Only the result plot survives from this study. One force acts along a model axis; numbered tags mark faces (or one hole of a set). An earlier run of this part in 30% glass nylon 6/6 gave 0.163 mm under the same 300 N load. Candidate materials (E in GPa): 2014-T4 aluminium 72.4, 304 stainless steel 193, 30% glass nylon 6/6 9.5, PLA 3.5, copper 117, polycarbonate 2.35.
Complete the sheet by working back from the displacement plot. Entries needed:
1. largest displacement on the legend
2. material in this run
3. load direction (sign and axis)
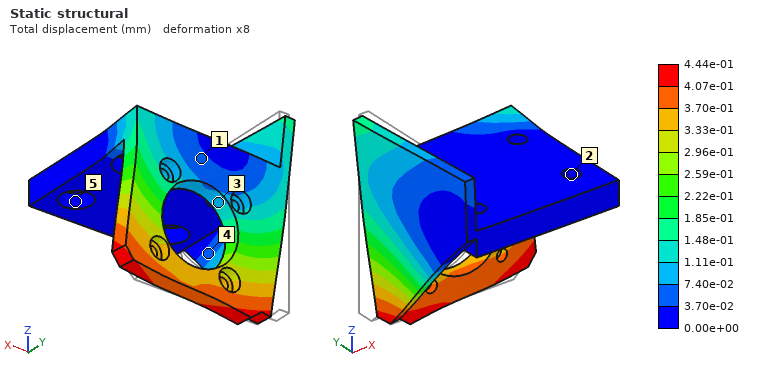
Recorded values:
4.44e-01 mm
PLA
+X
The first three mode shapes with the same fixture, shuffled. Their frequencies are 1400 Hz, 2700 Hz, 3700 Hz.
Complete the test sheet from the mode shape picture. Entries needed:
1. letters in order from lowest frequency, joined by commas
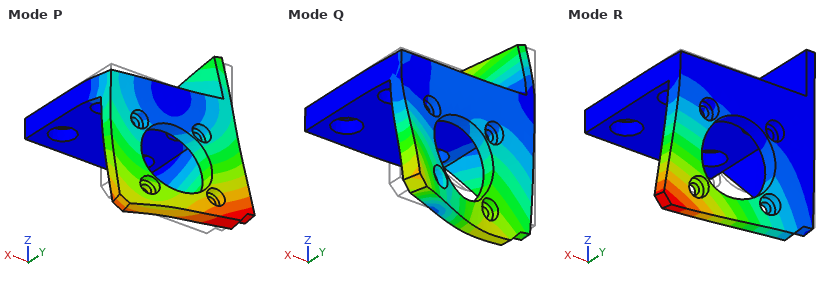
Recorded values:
R, P, Q
